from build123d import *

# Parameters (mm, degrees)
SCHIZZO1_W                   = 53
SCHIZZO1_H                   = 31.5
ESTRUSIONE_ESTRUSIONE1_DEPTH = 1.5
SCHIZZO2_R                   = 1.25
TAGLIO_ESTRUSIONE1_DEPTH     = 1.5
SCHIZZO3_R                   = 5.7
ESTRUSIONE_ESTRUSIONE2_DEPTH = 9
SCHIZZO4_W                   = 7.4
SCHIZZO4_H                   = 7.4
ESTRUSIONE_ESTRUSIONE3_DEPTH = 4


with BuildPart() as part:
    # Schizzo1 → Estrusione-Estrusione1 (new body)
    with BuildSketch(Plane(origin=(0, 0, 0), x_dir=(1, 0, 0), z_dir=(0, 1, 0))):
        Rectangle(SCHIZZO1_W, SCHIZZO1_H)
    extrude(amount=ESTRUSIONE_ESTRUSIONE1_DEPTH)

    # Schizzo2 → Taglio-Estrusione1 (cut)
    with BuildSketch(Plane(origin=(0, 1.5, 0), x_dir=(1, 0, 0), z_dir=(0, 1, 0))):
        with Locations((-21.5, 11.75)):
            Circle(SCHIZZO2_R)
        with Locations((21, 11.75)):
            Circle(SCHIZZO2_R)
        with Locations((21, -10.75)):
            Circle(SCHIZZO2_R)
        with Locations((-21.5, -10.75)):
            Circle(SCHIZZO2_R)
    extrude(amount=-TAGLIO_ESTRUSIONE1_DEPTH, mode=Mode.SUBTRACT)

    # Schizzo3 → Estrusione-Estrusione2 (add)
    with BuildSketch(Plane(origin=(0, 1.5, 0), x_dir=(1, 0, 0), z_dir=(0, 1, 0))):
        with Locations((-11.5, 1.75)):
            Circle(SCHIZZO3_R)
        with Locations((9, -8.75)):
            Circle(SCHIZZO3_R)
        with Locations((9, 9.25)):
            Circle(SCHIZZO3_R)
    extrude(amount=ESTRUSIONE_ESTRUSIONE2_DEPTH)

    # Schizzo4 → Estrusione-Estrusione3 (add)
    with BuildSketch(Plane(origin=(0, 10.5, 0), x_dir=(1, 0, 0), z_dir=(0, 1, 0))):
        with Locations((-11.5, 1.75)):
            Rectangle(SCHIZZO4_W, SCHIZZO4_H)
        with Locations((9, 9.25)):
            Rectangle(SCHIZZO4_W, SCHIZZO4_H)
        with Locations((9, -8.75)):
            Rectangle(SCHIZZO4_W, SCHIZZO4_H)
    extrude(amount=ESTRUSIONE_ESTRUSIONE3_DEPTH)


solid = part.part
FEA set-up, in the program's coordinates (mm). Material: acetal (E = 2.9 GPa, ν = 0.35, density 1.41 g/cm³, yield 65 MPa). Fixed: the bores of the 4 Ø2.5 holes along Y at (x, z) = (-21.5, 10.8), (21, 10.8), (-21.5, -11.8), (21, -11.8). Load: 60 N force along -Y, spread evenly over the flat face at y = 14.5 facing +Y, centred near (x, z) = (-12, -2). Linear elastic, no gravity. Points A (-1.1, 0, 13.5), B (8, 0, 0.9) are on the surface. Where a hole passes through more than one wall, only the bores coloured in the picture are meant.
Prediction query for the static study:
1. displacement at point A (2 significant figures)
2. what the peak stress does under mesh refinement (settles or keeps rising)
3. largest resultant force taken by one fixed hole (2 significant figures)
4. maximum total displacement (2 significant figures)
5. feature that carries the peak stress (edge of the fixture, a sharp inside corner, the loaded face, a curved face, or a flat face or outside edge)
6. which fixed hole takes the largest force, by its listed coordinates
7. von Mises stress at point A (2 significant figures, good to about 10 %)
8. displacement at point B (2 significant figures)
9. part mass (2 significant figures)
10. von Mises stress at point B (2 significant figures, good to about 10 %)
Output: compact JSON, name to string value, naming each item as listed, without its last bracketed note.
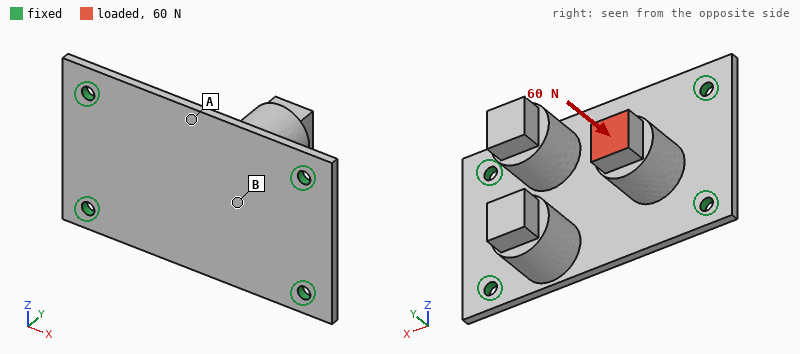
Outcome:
{"displacement at point A": "0.38 mm", "what the peak stress does under mesh refinement": "keeps rising", "largest resultant force taken by one fixed hole": "28 N", "maximum total displacement": "0.61 mm", "feature that carries the peak stress": "edge of the fixture", "which fixed hole takes the largest force, by its listed coordinates": "(-21.5, -11.8)", "von Mises stress at point A": "8.3 MPa", "displacement at point B": "0.31 mm", "part mass": "8.3 g", "von Mises stress at point B": "3.3 MPa"}
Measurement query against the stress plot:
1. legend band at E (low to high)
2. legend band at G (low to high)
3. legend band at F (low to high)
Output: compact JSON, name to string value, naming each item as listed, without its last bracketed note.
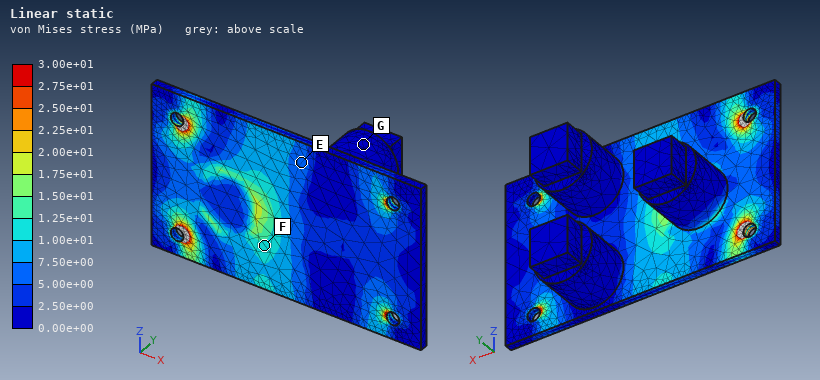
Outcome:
{"legend band at E": "5.00e+00 to 7.50e+00 MPa", "legend band at G": "0.00e+00 to 2.50e+00 MPa", "legend band at F": "1.00e+01 to 1.25e+01 MPa"}
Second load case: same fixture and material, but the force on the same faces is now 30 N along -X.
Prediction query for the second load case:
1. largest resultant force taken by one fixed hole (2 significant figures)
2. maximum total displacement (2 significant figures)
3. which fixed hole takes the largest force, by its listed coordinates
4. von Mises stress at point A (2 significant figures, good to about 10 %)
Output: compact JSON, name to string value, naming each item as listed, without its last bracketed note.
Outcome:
{"largest resultant force taken by one fixed hole": "12 N", "maximum total displacement": "0.60 mm", "which fixed hole takes the largest force, by its listed coordinates": "(-21.5, -11.8)", "von Mises stress at point A": "7.1 MPa"}
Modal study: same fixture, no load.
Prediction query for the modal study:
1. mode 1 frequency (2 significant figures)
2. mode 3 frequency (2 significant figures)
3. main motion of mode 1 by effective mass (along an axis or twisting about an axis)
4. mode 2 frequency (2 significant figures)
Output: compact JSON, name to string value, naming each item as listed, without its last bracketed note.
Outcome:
{"mode 1 frequency": "680 Hz", "mode 3 frequency": "1300 Hz", "main motion of mode 1 by effective mass": "along Y", "mode 2 frequency": "1100 Hz"}
